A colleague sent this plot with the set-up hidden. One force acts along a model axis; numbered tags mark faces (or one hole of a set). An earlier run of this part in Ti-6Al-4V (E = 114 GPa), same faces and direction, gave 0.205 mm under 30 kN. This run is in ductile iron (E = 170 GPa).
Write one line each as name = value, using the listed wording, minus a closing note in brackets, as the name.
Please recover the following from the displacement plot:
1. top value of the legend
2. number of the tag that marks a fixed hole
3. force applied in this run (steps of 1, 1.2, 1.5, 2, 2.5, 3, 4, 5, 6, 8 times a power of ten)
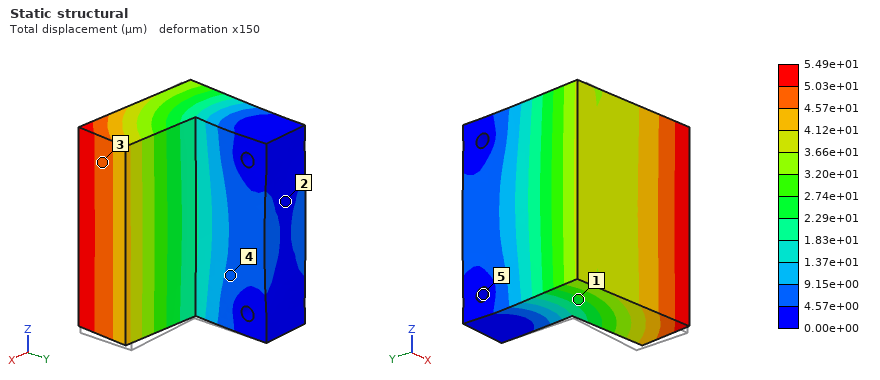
top value of the legend = 5.49e+01 µm
number of the tag that marks a fixed hole = 5
force applied in this run = 12 kN
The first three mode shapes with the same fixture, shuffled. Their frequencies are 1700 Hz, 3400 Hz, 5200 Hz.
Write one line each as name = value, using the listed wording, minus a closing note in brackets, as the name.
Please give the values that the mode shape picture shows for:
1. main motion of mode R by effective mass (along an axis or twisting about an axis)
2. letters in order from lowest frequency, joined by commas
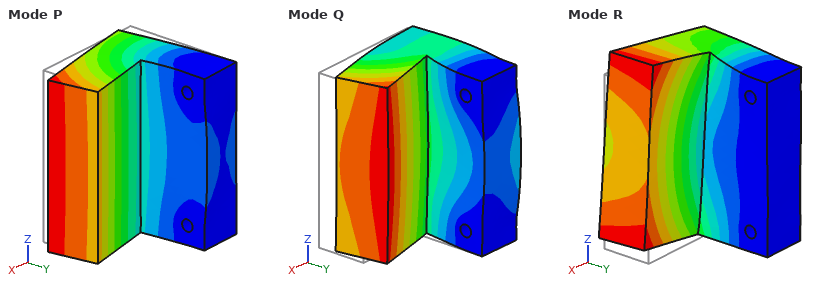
main motion of mode R by effective mass = along Z
letters in order from lowest frequency, joined by commas = P, R, Q
